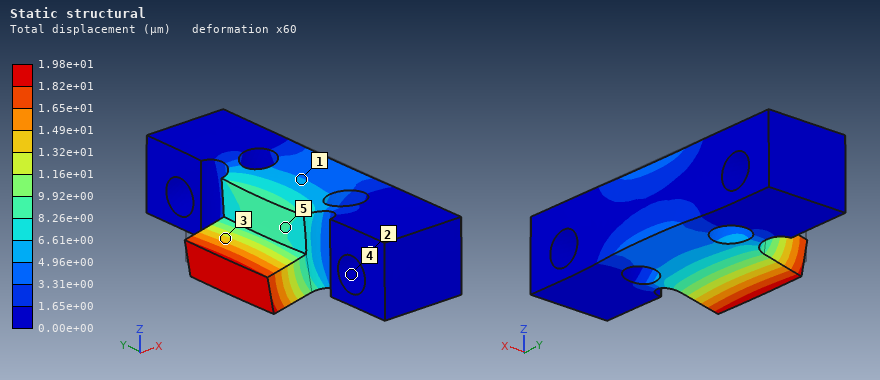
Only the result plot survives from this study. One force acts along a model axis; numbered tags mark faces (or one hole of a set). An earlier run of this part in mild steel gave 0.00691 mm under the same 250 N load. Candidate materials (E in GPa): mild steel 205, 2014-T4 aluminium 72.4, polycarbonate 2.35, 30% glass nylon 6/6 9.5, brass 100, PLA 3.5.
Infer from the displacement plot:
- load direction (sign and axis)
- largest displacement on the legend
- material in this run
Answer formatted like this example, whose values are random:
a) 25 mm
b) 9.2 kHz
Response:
a) -Z
b) 1.98e+01 µm
c) 2014-T4 aluminium
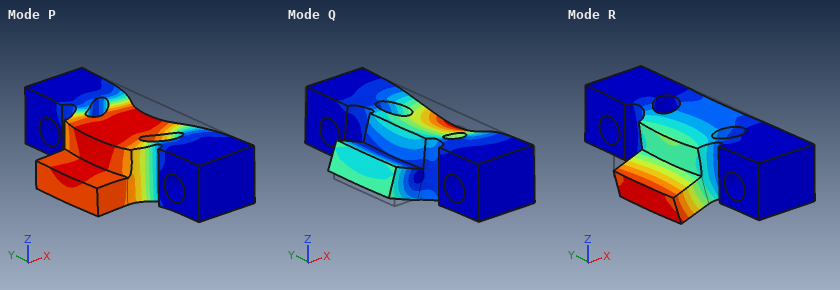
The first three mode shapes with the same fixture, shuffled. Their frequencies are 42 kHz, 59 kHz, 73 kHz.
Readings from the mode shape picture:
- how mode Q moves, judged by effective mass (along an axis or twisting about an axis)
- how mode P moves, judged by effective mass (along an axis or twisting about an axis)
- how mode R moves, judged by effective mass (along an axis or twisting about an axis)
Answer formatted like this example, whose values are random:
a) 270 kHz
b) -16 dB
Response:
a) along Z
b) along X
c) along Z
